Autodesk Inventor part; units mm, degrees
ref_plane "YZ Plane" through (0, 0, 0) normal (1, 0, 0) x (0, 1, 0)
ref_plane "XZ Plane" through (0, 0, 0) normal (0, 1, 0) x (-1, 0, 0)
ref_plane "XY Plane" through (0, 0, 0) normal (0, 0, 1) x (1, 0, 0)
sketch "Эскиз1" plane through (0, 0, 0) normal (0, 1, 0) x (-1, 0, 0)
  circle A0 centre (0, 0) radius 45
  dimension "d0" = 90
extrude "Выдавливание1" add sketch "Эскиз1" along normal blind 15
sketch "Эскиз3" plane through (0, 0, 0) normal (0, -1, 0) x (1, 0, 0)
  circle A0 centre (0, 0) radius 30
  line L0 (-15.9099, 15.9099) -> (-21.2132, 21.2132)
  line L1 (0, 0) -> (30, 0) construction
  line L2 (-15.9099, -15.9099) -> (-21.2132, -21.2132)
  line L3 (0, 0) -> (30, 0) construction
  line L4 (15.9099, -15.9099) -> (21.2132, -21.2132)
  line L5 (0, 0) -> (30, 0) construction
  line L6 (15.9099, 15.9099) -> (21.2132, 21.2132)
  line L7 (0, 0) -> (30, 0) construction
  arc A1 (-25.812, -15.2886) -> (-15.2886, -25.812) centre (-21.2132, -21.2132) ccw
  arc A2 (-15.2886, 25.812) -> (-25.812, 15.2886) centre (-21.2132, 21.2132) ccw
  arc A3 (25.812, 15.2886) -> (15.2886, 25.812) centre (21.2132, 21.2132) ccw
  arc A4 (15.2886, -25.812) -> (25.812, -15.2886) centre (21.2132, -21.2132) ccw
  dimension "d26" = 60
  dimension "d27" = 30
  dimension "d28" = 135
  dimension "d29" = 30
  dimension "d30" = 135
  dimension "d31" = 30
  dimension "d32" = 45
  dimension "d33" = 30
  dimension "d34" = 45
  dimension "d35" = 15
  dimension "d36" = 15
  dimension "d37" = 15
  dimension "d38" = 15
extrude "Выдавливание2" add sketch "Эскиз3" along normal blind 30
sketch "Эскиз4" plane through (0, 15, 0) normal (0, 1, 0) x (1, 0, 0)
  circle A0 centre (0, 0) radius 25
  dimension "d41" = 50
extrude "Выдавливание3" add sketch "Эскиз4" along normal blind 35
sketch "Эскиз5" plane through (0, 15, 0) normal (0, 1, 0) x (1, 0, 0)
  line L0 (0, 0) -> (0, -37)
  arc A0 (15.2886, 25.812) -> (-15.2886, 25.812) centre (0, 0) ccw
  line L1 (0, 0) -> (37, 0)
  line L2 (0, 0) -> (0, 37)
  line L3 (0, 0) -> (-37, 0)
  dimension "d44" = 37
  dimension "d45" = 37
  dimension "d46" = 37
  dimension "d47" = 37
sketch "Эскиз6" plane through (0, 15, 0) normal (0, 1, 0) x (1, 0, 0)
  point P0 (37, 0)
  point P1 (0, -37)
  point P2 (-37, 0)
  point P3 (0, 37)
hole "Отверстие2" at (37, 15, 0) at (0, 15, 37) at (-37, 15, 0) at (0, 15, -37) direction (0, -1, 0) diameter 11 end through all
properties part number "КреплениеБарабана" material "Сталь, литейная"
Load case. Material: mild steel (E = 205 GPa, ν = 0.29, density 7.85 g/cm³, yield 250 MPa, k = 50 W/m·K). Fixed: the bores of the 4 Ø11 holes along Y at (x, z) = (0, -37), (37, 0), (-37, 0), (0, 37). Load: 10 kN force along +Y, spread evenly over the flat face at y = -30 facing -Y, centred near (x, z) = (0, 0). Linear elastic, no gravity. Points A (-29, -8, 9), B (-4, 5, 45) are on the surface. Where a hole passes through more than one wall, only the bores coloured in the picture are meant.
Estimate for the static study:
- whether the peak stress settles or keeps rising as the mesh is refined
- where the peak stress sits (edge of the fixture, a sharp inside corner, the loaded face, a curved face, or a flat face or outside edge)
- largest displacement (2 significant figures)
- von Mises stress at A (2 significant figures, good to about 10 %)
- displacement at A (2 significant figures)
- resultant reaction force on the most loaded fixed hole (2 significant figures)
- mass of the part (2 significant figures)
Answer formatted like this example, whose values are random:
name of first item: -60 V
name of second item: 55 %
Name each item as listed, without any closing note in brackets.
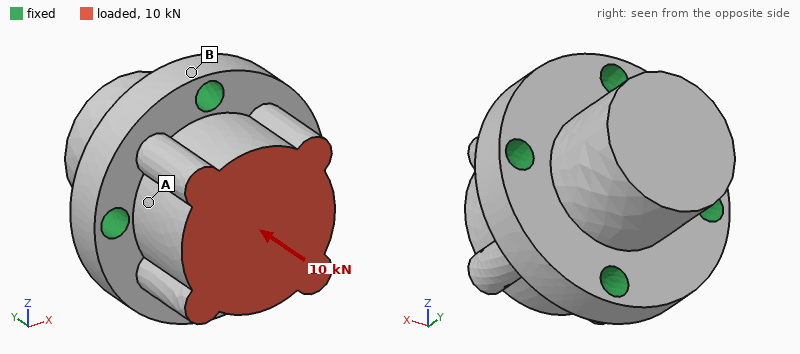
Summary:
whether the peak stress settles or keeps rising as the mesh is refined: keeps rising
where the peak stress sits: edge of the fixture
largest displacement: 1.3 µm
von Mises stress at A: 4.6 MPa
displacement at A: 0.94 µm
resultant reaction force on the most loaded fixed hole: 2.6 kN
mass of the part: 2.0 kg
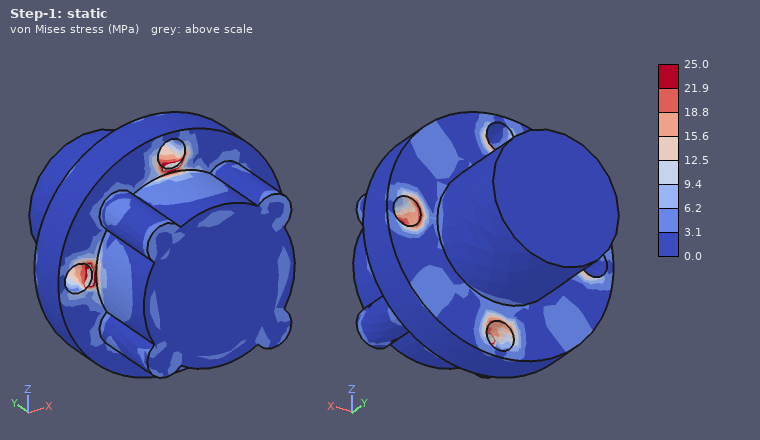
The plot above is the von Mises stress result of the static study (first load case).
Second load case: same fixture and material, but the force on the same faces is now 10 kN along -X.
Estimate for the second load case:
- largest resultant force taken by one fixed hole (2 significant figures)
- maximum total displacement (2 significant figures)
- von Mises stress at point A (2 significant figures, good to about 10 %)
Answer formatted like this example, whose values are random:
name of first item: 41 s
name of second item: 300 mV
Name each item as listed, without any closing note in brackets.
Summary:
largest resultant force taken by one fixed hole: 6.1 kN
maximum total displacement: 5.3 µm
von Mises stress at point A: 11 MPa
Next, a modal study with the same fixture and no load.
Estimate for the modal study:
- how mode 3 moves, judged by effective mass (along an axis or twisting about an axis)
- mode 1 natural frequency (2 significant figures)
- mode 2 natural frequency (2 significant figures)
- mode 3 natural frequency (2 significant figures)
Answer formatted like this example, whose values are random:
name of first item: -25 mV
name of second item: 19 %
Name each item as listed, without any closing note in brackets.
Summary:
how mode 3 moves, judged by effective mass: along Y
mode 1 natural frequency: 9700 Hz
mode 2 natural frequency: 9700 Hz
mode 3 natural frequency: 12 kHz
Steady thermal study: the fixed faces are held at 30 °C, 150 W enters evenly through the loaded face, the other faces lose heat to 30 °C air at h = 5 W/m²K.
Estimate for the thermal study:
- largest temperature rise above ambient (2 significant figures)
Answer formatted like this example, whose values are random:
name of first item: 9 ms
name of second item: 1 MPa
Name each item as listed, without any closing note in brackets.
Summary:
largest temperature rise above ambient: 47 K
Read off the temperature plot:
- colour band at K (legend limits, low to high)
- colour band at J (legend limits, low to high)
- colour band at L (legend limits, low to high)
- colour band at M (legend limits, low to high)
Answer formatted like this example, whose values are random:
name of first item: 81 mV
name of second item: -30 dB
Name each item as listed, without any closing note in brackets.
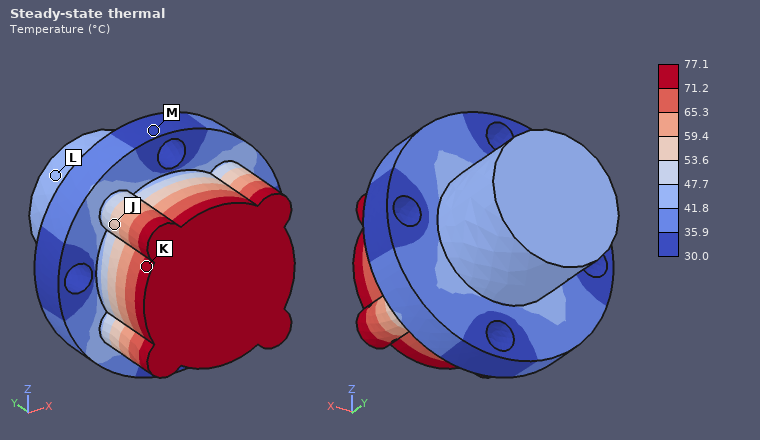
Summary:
colour band at K: 71.2 to 77.1 °C
colour band at J: 53.6 to 59.4 °C
colour band at L: 41.8 to 47.7 °C
colour band at M: 30.0 to 35.9 °C
